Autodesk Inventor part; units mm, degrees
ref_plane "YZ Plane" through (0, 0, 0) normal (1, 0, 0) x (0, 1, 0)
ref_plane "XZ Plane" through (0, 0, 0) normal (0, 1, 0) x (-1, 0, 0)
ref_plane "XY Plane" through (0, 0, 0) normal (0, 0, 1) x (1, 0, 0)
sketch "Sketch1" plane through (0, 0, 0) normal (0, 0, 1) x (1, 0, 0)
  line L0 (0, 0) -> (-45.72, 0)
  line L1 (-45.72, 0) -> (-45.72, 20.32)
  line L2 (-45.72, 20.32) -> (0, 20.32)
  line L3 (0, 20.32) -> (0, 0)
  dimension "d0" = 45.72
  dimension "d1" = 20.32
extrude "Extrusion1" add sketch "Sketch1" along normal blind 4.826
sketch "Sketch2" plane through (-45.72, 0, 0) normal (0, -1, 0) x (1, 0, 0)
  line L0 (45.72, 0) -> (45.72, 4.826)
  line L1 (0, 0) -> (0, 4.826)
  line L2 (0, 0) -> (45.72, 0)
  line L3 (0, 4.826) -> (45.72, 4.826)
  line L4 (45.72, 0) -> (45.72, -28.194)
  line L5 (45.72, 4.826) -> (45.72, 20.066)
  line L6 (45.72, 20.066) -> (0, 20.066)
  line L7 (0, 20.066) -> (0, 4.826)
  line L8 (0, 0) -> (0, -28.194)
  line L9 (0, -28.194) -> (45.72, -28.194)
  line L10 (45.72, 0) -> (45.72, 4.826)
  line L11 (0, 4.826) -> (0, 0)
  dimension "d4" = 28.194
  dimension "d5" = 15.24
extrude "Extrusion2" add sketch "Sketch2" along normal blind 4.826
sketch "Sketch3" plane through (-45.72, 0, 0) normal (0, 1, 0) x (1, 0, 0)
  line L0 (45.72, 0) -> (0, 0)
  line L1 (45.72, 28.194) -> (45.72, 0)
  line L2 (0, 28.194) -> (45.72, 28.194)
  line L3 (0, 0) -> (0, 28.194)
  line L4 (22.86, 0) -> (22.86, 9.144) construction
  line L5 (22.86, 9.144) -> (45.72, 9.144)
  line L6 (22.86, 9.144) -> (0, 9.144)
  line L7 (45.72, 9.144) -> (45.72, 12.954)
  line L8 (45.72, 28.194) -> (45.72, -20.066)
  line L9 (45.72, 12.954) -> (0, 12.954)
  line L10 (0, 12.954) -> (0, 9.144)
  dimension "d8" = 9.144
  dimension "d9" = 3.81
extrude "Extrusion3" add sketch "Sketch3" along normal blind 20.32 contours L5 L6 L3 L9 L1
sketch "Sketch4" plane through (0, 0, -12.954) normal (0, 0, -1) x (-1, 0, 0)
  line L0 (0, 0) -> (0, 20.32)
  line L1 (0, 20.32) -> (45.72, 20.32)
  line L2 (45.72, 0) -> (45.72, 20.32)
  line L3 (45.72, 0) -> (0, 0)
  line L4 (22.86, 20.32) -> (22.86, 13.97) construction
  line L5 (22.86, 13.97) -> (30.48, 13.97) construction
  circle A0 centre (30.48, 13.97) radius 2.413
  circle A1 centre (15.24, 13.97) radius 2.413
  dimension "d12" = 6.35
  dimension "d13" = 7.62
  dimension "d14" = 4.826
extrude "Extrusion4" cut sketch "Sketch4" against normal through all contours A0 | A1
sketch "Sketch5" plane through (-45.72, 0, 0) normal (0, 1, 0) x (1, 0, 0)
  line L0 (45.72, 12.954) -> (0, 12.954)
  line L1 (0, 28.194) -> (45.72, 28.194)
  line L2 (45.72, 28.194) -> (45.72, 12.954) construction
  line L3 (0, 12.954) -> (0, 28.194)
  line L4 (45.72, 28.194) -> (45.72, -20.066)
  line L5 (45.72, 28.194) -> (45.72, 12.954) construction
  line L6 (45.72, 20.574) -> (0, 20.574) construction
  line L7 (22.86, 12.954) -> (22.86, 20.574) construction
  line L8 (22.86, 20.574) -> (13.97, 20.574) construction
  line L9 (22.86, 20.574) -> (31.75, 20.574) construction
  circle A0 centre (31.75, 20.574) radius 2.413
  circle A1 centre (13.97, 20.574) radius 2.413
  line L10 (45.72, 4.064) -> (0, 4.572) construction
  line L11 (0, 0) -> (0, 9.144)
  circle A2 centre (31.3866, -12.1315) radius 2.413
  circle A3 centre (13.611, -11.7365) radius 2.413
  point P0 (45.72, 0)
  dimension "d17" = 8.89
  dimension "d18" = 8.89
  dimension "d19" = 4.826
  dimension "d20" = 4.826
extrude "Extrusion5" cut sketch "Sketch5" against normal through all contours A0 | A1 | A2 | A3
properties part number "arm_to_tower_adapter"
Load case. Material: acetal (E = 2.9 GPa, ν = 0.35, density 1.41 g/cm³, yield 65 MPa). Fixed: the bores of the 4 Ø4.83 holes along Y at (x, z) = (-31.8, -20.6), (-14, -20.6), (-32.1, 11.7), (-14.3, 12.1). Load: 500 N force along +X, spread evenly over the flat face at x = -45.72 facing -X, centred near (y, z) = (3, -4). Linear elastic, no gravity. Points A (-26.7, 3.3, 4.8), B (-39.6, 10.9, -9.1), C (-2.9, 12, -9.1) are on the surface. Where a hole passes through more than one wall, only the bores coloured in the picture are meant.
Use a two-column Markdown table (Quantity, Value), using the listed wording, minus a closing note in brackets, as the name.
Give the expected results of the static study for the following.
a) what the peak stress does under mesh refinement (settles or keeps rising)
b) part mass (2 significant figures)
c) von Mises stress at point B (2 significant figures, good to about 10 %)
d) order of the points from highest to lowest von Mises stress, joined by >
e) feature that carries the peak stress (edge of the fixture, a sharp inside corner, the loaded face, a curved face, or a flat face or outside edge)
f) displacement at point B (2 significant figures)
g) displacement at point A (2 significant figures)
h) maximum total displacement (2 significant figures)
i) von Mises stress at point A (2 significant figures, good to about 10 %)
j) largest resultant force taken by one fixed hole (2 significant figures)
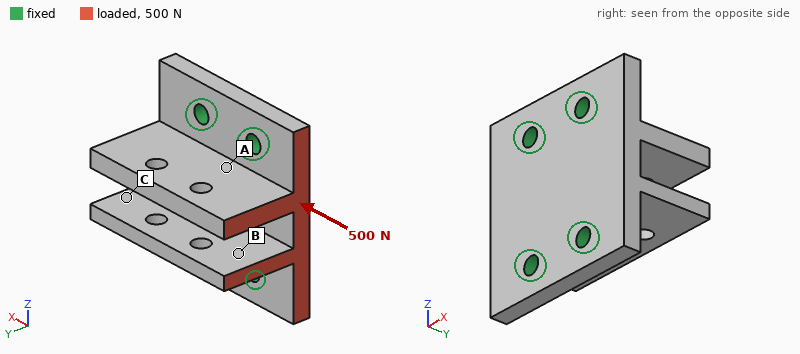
| Quantity | Value |
|---|---|
| what the peak stress does under mesh refinement | keeps rising |
| part mass | 25 g |
| von Mises stress at point B | 1.3 MPa |
| order of the points from highest to lowest von Mises stress, joined by > | A > B > C |
| feature that carries the peak stress | edge of the fixture |
| displacement at point B | 53 µm |
| displacement at point A | 22 µm |
| maximum total displacement | 84 µm |
| von Mises stress at point A | 2.4 MPa |
| largest resultant force taken by one fixed hole | 180 N |
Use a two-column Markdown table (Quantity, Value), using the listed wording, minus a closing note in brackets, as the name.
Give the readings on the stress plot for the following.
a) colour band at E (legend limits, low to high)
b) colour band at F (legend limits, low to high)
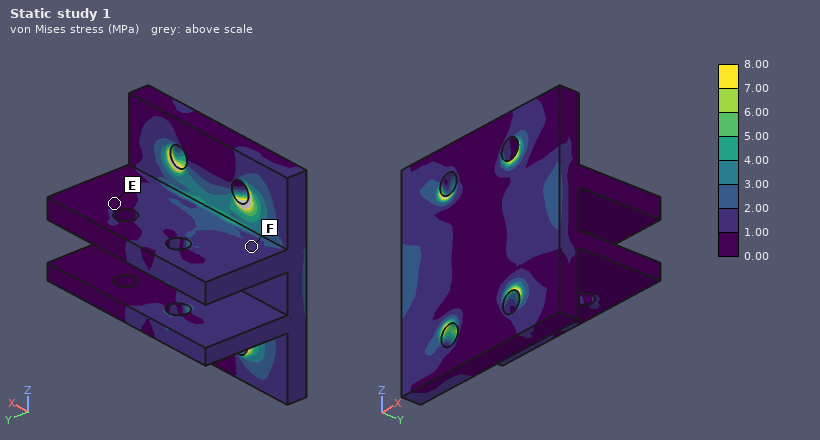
| Quantity | Value |
|---|---|
| colour band at E | 0.00 to 1.00 MPa |
| colour band at F | 1.00 to 2.00 MPa |
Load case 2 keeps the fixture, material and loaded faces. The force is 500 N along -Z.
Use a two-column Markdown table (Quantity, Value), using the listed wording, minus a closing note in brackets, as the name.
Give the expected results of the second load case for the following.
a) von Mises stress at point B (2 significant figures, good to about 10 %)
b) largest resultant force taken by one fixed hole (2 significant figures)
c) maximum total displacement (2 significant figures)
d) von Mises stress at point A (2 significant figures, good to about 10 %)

| Quantity | Value |
|---|---|
| von Mises stress at point B | 9.7 MPa |
| largest resultant force taken by one fixed hole | 310 N |
| maximum total displacement | 0.63 mm |
| von Mises stress at point A | 5.6 MPa |
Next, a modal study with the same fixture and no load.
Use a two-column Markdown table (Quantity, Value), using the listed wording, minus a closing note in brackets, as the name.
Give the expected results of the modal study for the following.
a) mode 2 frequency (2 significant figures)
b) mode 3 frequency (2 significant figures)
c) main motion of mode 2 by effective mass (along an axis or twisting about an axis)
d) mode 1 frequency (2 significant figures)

| Quantity | Value |
|---|---|
| mode 2 frequency | 2100 Hz |
| mode 3 frequency | 2300 Hz |
| main motion of mode 2 by effective mass | along Z |
| mode 1 frequency | 1700 Hz |
